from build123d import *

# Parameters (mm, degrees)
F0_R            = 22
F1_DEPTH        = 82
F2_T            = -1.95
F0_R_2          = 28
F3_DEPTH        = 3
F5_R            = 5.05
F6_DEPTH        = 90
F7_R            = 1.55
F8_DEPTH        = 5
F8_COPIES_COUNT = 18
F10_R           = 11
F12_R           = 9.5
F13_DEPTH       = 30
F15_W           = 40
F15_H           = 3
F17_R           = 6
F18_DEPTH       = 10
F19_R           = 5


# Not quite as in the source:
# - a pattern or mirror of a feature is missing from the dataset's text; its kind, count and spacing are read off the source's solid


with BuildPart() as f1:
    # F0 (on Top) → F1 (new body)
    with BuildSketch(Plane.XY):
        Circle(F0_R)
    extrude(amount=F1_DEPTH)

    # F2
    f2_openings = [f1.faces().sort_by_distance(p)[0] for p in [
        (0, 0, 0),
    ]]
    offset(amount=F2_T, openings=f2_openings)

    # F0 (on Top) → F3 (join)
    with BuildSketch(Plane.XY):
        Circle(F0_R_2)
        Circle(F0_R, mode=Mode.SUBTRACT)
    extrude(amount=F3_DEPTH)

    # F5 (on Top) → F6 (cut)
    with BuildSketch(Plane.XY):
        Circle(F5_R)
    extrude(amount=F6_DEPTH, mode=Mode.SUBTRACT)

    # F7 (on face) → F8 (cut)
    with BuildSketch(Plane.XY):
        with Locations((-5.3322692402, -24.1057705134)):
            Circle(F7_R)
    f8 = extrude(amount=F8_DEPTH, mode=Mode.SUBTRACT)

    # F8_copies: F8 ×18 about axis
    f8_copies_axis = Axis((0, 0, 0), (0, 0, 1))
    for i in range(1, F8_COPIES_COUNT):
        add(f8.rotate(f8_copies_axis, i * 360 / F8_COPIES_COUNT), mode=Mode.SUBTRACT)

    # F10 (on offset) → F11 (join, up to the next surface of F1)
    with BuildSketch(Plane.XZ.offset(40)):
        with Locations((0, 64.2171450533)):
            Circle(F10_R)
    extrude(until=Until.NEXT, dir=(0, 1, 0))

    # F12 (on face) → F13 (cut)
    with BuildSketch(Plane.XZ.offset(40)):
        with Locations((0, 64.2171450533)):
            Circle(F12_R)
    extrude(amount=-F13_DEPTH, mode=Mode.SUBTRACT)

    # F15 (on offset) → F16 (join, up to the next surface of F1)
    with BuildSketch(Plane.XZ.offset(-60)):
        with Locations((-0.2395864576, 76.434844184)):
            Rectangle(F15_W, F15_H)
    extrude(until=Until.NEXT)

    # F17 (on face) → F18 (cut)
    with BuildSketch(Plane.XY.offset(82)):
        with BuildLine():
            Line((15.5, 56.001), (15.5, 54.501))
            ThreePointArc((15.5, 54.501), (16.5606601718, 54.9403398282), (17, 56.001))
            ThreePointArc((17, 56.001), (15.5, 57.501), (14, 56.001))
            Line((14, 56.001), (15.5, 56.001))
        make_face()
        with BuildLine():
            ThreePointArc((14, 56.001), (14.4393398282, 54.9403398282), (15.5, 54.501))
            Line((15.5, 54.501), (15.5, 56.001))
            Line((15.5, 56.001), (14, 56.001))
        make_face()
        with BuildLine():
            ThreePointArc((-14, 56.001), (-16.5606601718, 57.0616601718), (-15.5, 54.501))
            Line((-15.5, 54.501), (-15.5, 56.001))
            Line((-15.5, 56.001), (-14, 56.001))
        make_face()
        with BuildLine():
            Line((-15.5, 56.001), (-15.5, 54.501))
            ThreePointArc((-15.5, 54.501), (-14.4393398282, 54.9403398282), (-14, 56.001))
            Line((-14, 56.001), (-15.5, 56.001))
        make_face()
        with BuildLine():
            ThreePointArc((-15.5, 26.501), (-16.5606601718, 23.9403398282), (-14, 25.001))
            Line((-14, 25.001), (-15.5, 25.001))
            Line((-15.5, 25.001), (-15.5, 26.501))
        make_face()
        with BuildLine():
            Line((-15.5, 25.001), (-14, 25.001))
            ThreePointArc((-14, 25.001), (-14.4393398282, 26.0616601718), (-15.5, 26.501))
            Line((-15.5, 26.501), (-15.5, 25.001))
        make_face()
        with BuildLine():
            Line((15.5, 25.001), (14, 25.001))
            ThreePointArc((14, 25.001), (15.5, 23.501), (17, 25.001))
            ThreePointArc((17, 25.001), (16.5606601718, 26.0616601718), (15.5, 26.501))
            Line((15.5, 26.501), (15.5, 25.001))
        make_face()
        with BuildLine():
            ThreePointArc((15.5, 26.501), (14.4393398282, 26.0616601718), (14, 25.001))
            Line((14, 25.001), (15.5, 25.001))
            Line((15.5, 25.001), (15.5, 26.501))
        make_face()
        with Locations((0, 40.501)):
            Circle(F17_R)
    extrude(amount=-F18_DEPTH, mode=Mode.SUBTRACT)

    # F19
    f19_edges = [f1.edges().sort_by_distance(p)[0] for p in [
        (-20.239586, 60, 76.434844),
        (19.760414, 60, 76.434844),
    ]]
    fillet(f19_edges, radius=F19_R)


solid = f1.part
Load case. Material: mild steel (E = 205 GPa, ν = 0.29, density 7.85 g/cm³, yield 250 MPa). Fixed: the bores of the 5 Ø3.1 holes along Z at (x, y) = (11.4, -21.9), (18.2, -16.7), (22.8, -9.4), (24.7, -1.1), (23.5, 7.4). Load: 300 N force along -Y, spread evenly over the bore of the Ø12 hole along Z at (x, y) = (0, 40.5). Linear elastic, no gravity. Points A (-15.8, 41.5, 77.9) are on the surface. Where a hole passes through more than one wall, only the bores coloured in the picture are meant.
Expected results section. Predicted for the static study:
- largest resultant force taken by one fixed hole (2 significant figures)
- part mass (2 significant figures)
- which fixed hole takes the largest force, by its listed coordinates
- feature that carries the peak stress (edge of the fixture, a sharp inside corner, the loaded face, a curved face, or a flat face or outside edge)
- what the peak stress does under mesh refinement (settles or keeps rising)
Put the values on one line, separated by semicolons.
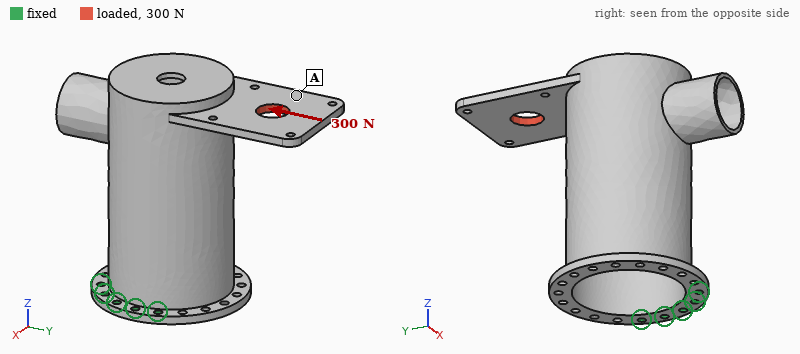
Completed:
1.2 kN; 250 g; (23.5, 7.4); edge of the fixture; keeps rising
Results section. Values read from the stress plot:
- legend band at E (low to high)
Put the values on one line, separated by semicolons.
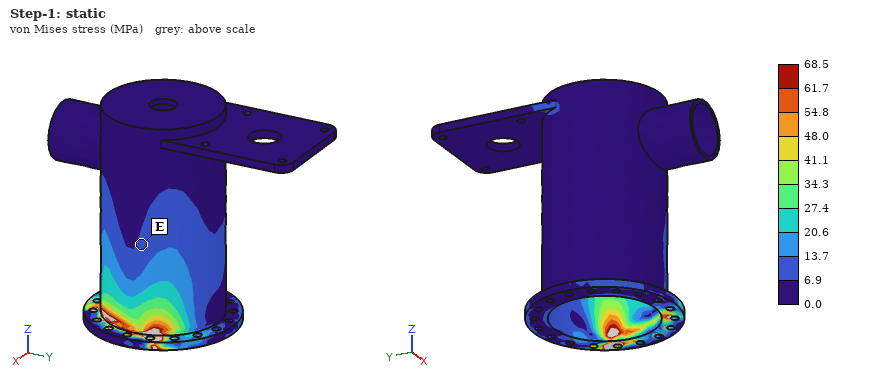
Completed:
6.9 to 13.7 MPa
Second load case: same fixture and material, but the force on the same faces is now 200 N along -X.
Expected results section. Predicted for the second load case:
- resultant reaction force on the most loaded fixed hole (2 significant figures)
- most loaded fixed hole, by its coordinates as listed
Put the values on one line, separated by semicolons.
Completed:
1.1 kN; (11.4, -21.9)
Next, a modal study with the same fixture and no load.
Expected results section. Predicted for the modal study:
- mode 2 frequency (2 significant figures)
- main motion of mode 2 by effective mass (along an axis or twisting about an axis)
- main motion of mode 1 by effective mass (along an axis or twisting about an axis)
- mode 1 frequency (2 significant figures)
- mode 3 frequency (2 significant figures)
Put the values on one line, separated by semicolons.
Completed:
1100 Hz; along Y; along X; 420 Hz; 1400 Hz
